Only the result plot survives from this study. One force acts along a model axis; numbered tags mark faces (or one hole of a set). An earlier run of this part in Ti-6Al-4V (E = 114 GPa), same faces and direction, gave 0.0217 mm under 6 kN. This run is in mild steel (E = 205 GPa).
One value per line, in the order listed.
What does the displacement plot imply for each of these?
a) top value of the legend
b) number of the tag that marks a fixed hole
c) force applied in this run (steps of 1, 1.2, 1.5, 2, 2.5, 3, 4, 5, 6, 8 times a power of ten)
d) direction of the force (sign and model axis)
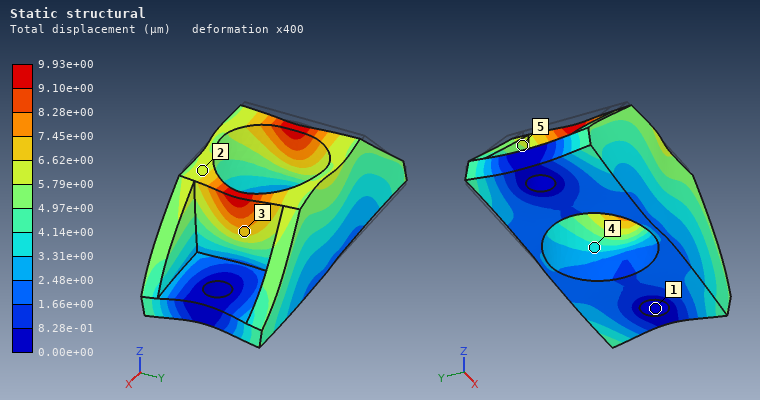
9.93e+00 µm
1
5 kN
+X
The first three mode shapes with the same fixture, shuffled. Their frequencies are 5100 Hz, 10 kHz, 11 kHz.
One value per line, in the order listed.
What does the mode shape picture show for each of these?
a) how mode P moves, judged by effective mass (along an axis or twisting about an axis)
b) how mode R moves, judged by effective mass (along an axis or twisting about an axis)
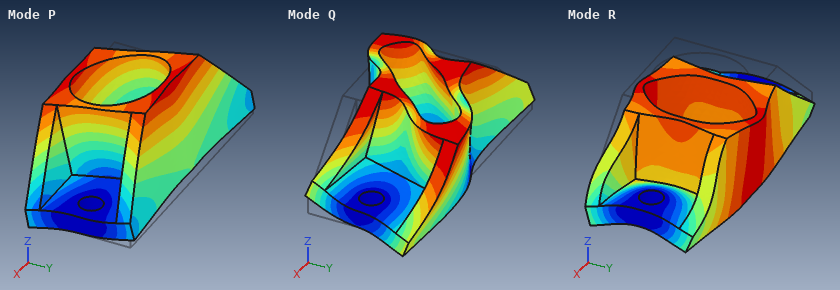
along Y
along Z
